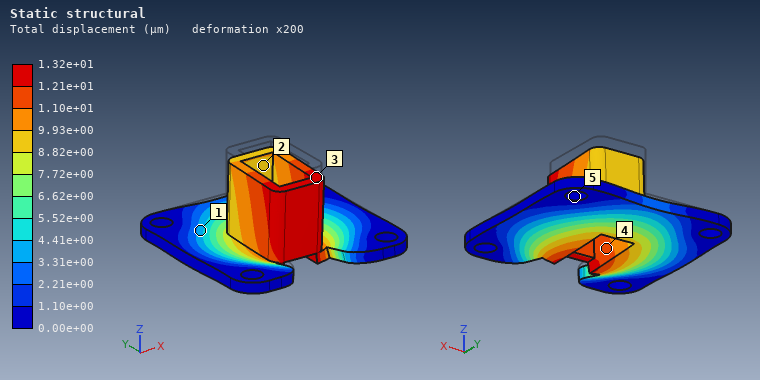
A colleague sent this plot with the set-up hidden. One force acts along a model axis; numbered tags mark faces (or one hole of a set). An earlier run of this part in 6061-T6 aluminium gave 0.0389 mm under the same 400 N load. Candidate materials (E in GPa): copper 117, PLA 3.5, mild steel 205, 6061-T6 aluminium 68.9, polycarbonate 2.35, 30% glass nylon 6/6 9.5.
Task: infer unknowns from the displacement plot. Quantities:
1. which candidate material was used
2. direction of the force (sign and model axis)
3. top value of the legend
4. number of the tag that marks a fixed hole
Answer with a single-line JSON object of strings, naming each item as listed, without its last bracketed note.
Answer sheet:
{"which candidate material was used": "mild steel", "direction of the force": "-Z", "top value of the legend": "1.32e+01 µm", "number of the tag that marks a fixed hole": "5"}
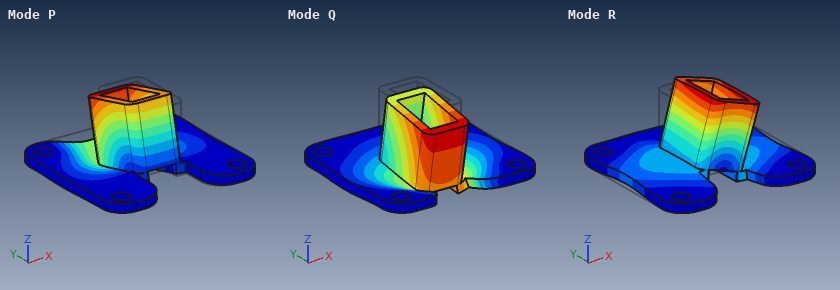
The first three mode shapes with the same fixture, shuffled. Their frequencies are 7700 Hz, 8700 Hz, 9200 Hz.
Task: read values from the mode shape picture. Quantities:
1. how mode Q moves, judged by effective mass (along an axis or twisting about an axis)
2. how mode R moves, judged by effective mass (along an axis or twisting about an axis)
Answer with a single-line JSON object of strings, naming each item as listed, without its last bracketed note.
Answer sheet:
{"how mode Q moves, judged by effective mass": "along Z", "how mode R moves, judged by effective mass": "along X"}
